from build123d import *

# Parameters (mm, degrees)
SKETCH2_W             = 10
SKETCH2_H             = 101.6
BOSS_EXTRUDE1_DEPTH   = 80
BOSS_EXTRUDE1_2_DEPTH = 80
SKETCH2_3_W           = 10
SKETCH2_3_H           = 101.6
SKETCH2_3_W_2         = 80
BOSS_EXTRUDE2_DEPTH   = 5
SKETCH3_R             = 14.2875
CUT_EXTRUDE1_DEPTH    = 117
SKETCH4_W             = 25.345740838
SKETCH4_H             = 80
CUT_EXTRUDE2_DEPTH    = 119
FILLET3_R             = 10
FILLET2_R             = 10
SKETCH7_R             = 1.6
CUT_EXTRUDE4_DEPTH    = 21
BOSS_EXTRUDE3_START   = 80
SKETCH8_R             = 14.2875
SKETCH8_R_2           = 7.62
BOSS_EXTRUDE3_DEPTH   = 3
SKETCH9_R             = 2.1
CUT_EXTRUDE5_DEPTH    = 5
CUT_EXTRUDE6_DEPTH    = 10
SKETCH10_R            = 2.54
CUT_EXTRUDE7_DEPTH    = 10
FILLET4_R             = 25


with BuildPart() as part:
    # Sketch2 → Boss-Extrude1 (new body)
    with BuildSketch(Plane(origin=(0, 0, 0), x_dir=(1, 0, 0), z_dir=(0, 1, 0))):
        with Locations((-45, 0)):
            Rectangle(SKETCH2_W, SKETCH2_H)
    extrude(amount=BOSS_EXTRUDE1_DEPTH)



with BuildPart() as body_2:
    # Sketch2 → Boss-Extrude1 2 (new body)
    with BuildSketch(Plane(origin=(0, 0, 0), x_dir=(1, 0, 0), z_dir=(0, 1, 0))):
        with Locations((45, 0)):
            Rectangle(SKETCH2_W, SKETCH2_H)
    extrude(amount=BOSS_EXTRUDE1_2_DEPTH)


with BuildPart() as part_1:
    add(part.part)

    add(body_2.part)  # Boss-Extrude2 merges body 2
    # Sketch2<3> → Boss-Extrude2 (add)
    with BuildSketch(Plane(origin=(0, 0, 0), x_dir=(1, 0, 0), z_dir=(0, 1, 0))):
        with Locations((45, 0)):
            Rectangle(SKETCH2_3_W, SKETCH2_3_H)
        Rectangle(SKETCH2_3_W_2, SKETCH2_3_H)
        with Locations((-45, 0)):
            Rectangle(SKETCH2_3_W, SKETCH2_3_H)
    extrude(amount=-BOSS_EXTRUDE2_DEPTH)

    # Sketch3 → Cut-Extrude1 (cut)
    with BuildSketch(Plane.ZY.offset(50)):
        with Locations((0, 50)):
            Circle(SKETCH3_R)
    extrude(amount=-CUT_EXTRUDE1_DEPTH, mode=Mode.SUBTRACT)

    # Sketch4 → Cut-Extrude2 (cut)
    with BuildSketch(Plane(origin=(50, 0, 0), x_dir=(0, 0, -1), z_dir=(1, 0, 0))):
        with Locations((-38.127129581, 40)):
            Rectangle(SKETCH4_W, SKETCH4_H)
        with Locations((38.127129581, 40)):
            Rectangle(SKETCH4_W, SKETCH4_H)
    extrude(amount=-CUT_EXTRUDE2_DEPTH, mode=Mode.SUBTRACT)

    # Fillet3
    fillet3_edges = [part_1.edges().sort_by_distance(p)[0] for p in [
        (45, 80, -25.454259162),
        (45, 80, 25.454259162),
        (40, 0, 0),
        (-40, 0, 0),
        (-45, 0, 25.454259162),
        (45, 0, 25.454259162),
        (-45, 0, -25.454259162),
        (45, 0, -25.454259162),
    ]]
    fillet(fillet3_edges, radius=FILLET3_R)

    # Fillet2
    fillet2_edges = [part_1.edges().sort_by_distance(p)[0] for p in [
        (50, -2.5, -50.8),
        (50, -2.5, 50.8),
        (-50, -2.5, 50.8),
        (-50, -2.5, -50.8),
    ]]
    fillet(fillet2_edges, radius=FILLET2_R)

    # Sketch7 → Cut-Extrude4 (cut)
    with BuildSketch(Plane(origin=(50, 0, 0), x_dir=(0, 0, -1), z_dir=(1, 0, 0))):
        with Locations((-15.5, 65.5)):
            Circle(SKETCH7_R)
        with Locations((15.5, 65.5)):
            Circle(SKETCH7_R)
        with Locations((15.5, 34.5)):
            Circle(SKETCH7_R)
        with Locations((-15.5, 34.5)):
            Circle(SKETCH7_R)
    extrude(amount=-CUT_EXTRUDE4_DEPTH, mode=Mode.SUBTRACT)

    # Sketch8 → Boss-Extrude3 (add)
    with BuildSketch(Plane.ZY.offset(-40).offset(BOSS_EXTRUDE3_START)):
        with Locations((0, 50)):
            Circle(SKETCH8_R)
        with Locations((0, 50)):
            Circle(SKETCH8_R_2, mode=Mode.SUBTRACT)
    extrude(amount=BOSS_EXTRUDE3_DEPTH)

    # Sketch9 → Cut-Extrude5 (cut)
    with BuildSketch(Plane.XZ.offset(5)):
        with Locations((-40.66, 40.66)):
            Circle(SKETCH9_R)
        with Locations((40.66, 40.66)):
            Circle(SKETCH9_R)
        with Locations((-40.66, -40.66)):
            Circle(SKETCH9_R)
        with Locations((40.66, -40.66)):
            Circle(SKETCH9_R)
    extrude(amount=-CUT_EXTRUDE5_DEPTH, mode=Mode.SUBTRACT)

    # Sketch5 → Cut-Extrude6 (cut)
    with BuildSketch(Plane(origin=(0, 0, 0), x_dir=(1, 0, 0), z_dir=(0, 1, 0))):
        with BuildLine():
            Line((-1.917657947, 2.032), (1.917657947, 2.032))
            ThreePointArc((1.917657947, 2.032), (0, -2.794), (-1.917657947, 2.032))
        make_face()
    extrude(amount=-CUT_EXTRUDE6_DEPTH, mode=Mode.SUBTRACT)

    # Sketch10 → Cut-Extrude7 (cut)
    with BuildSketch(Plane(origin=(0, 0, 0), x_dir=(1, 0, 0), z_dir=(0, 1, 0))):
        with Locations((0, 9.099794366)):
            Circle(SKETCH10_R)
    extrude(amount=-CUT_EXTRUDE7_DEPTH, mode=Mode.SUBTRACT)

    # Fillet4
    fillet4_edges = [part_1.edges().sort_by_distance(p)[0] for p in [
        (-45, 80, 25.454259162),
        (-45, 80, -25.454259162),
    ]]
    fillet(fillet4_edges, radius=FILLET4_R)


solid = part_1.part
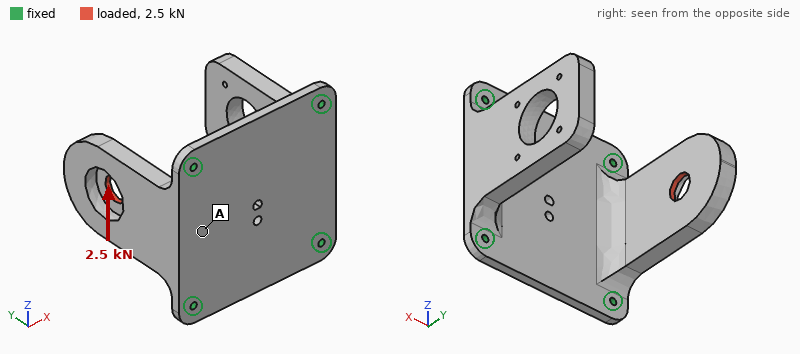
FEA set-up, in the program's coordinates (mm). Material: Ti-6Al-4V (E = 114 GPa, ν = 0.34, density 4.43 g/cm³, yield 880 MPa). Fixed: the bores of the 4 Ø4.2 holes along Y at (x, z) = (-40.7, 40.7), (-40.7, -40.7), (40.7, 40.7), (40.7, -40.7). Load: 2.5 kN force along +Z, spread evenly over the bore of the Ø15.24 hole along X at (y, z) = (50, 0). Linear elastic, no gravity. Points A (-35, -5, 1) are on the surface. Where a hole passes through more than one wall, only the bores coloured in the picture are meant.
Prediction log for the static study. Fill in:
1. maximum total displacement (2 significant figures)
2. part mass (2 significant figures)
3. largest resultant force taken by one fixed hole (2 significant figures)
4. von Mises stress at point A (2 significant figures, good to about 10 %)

96 µm
530 g
2.2 kN
11 MPa
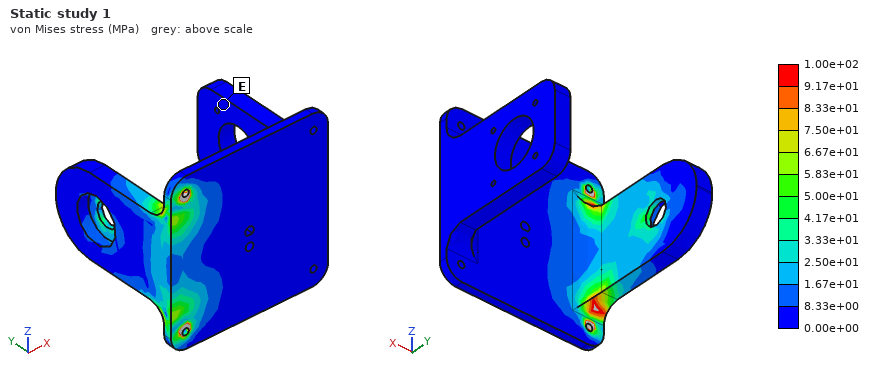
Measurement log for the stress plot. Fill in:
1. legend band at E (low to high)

0.00e+00 to 8.33e+00 MPa
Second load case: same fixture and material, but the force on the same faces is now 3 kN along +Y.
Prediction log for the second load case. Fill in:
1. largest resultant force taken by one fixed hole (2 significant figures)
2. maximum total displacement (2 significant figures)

1.9 kN
36 µm
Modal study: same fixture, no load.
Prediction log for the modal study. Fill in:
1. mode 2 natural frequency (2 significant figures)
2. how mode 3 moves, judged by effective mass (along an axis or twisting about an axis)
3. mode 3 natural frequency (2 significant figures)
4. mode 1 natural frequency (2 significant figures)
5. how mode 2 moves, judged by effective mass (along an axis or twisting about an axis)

910 Hz
along Z
2800 Hz
750 Hz
along X
